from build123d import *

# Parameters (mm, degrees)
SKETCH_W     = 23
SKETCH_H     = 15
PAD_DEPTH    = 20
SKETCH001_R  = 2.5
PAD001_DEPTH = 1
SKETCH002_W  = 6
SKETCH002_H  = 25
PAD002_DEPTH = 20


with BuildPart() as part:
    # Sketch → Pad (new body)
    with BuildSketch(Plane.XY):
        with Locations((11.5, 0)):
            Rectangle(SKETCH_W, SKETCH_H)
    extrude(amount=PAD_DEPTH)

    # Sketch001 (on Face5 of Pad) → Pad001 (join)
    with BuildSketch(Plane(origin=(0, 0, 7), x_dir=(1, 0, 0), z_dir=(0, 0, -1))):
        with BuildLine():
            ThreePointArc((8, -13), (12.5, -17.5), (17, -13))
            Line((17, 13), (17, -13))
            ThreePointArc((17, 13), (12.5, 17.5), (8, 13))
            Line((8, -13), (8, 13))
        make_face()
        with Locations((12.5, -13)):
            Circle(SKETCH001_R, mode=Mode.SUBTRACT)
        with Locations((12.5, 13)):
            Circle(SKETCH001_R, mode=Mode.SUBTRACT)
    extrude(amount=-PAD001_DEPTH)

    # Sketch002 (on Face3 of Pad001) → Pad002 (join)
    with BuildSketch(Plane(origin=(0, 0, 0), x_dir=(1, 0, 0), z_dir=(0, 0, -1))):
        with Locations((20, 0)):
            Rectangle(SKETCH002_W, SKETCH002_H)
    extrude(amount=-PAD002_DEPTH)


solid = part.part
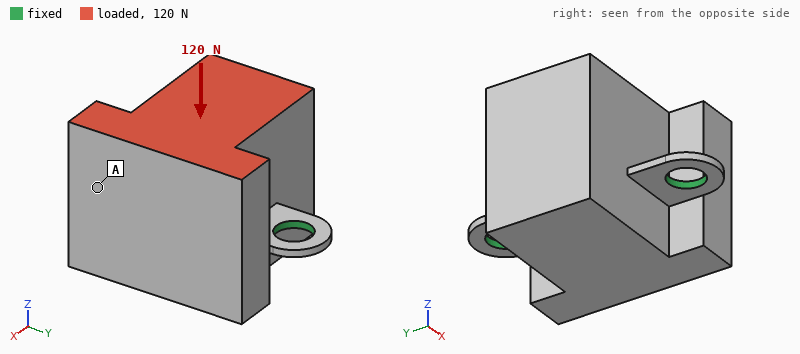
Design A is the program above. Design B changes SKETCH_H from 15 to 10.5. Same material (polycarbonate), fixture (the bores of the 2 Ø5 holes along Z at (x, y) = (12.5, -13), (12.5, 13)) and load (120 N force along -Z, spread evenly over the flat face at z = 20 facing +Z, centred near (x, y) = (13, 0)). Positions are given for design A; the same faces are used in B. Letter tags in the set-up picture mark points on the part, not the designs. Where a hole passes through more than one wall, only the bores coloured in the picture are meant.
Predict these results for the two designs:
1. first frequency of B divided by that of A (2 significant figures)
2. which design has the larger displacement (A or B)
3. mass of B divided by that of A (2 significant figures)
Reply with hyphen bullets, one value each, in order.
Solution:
- 0.80
- B
- 0.82
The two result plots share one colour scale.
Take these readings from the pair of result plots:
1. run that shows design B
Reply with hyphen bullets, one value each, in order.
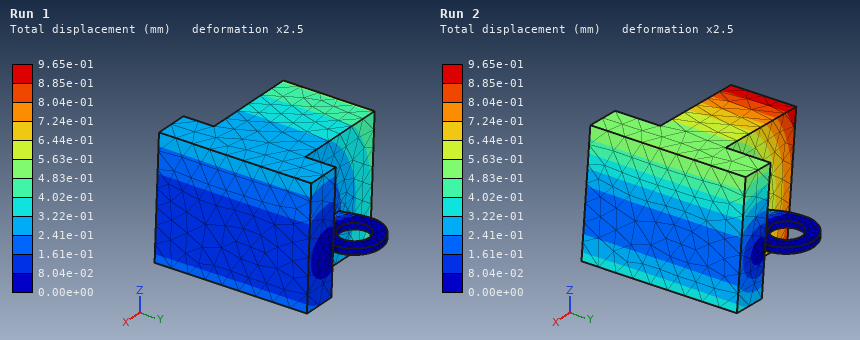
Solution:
- Run 2
